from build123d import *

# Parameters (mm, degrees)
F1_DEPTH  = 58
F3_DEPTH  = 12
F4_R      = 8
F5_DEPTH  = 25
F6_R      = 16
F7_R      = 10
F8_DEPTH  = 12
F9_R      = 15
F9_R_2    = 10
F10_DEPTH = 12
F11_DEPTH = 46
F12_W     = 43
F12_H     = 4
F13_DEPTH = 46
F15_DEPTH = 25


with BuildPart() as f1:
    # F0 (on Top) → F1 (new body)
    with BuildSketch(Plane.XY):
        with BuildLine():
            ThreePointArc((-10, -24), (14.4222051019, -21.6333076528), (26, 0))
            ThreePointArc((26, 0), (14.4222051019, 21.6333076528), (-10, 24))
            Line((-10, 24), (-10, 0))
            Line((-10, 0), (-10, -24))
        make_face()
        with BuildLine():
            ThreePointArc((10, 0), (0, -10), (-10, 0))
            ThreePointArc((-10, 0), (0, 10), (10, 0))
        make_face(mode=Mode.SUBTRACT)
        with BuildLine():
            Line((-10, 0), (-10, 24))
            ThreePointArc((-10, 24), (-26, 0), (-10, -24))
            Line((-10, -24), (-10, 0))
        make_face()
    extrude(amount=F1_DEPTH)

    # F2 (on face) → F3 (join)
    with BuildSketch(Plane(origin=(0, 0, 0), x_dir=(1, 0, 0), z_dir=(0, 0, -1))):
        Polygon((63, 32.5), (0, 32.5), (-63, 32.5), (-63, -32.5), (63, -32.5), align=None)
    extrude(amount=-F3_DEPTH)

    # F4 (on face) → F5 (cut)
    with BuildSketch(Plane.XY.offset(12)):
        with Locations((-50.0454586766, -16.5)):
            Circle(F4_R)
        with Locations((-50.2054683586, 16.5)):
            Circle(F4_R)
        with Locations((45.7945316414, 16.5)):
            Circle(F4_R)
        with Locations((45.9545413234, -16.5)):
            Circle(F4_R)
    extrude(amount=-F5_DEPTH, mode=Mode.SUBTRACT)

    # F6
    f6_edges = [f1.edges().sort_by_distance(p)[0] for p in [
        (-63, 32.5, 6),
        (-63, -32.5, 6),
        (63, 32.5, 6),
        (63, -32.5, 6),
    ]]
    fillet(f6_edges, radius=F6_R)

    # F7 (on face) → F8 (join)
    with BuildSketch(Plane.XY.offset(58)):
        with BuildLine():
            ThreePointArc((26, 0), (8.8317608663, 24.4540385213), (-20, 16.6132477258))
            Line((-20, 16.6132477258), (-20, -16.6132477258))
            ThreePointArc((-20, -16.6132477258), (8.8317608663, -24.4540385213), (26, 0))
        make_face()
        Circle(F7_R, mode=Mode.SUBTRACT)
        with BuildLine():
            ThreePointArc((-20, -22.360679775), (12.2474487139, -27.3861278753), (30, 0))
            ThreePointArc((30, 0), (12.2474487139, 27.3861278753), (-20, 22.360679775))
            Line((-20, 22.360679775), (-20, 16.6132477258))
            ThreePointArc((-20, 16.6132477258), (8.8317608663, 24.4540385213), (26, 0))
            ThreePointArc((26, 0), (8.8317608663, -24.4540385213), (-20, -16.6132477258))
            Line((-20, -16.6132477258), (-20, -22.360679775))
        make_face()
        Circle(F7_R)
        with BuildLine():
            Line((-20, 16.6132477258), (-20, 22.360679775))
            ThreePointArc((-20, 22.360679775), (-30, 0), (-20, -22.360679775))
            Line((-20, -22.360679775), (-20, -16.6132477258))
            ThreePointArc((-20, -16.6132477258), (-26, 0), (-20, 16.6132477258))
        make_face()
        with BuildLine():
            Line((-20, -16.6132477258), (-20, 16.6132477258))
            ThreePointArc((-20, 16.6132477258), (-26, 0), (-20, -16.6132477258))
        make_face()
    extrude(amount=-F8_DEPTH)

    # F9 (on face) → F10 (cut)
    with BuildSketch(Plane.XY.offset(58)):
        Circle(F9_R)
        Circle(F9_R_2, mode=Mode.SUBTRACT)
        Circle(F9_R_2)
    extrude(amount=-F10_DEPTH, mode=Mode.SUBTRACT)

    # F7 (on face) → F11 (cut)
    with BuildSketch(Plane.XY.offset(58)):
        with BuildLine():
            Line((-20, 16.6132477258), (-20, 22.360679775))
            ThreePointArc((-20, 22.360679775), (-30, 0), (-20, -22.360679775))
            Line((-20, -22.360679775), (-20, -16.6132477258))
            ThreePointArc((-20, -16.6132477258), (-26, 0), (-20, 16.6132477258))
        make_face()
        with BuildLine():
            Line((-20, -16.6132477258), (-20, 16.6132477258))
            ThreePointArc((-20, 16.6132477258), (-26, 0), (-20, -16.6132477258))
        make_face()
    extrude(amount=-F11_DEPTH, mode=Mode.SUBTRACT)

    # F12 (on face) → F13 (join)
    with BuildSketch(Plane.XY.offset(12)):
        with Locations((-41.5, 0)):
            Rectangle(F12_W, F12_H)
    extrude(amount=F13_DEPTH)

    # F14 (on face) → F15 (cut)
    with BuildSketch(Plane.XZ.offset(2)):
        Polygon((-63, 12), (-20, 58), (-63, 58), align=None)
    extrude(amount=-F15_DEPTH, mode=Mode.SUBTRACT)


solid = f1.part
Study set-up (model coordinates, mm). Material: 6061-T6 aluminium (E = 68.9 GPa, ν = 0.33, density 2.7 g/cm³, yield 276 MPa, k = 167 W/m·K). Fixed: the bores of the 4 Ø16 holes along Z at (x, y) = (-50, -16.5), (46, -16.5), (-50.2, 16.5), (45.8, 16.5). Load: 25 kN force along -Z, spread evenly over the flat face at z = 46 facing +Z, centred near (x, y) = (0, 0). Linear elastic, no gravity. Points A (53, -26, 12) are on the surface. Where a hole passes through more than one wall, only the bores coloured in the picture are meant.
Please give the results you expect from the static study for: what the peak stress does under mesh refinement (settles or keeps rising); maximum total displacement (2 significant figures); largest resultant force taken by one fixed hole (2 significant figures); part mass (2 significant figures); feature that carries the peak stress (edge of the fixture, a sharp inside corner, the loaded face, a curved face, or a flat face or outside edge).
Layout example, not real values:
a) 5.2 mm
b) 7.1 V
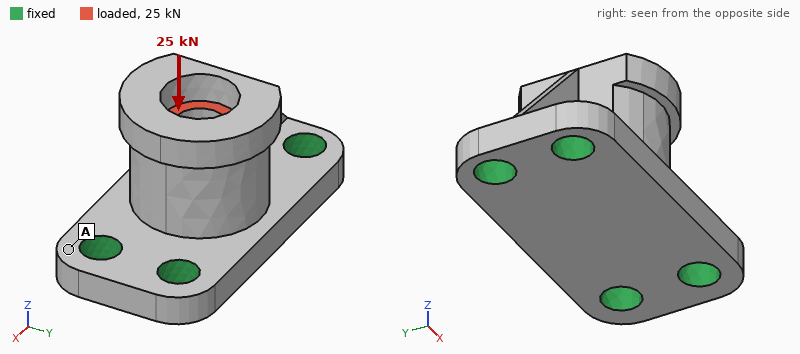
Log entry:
a) keeps rising
b) 60 µm
c) 7.4 kN
d) 460 g
e) edge of the fixture
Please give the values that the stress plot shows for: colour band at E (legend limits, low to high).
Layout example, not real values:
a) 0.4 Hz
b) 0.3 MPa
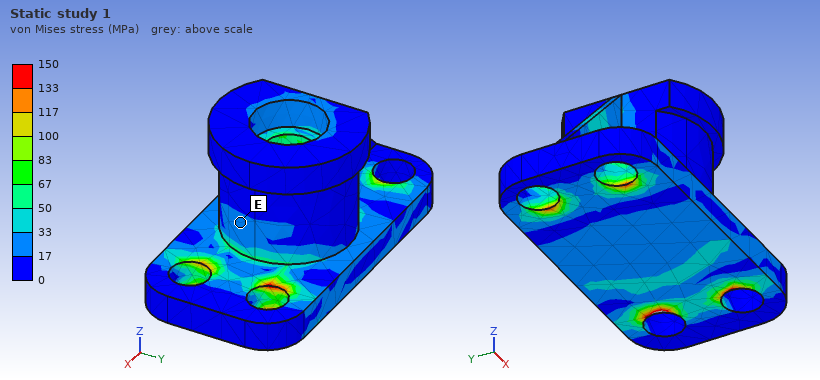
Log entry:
a) 17 to 33 MPa
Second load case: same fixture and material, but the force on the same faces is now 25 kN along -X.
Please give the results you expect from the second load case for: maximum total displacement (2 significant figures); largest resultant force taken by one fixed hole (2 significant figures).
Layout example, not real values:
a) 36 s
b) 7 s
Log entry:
a) 0.12 mm
b) 9.8 kN
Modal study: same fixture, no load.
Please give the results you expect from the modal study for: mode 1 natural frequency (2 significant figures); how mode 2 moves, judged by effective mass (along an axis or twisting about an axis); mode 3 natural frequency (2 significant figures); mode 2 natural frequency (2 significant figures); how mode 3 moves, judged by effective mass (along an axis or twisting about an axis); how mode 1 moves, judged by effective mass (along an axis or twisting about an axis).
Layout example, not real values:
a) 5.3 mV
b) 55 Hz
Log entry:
a) 3400 Hz
b) along Z
c) 7000 Hz
d) 6300 Hz
e) along X
f) along Y
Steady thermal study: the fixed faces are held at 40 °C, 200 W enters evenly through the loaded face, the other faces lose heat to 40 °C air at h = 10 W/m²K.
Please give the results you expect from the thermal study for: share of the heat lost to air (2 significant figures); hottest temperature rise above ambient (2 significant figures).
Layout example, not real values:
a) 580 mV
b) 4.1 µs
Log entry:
a) 3.3 %
b) 54 K
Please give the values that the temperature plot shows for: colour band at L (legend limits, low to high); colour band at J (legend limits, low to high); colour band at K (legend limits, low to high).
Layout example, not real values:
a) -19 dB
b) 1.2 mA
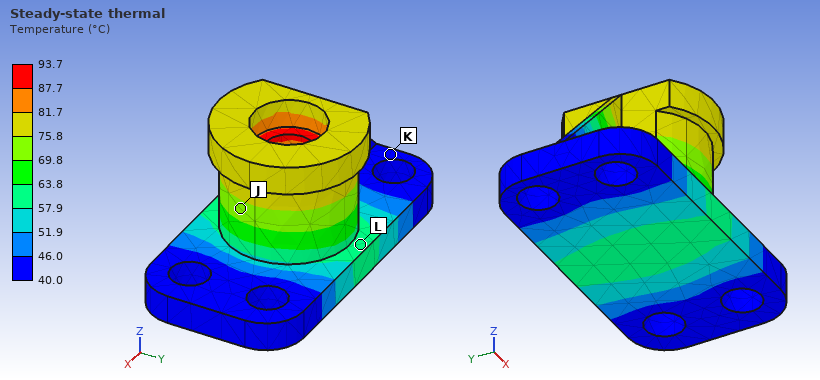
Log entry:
a) 57.9 to 63.8 °C
b) 69.8 to 75.8 °C
c) 40.0 to 46.0 °C
